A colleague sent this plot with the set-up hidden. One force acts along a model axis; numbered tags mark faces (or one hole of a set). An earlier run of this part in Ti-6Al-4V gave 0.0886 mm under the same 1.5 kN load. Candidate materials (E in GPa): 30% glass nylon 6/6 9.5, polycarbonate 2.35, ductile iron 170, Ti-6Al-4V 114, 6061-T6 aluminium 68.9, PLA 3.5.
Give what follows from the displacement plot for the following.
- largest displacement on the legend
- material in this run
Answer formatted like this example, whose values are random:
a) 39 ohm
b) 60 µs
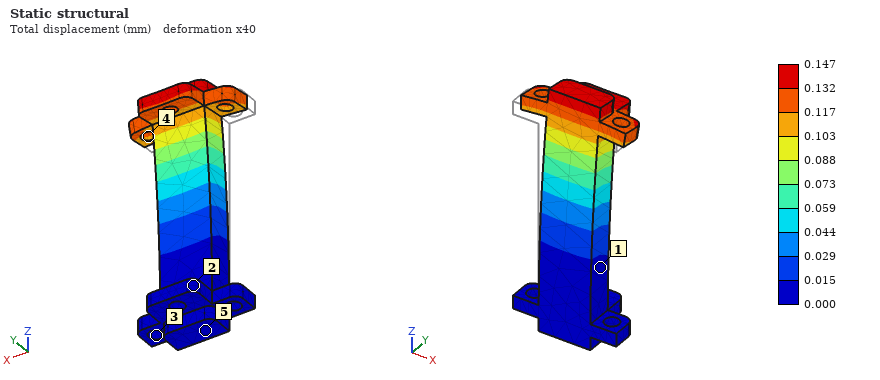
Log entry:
a) 0.147 mm
b) 6061-T6 aluminium
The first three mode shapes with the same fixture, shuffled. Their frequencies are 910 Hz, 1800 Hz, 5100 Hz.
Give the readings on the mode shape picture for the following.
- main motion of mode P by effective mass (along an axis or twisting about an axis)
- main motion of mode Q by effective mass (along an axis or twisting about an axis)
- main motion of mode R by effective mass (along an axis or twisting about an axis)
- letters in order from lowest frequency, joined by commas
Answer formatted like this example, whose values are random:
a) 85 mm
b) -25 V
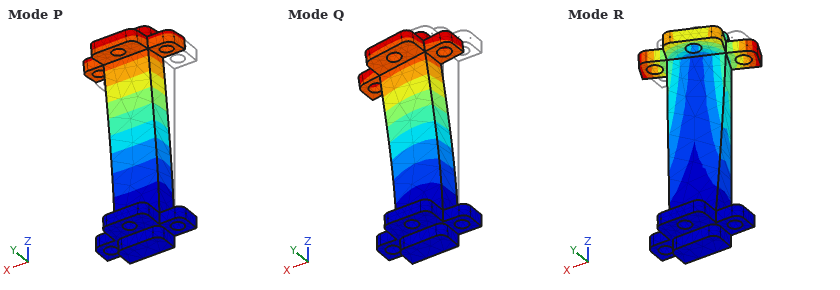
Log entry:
a) along Y
b) along X
c) twisting about Z
d) P, Q, R
